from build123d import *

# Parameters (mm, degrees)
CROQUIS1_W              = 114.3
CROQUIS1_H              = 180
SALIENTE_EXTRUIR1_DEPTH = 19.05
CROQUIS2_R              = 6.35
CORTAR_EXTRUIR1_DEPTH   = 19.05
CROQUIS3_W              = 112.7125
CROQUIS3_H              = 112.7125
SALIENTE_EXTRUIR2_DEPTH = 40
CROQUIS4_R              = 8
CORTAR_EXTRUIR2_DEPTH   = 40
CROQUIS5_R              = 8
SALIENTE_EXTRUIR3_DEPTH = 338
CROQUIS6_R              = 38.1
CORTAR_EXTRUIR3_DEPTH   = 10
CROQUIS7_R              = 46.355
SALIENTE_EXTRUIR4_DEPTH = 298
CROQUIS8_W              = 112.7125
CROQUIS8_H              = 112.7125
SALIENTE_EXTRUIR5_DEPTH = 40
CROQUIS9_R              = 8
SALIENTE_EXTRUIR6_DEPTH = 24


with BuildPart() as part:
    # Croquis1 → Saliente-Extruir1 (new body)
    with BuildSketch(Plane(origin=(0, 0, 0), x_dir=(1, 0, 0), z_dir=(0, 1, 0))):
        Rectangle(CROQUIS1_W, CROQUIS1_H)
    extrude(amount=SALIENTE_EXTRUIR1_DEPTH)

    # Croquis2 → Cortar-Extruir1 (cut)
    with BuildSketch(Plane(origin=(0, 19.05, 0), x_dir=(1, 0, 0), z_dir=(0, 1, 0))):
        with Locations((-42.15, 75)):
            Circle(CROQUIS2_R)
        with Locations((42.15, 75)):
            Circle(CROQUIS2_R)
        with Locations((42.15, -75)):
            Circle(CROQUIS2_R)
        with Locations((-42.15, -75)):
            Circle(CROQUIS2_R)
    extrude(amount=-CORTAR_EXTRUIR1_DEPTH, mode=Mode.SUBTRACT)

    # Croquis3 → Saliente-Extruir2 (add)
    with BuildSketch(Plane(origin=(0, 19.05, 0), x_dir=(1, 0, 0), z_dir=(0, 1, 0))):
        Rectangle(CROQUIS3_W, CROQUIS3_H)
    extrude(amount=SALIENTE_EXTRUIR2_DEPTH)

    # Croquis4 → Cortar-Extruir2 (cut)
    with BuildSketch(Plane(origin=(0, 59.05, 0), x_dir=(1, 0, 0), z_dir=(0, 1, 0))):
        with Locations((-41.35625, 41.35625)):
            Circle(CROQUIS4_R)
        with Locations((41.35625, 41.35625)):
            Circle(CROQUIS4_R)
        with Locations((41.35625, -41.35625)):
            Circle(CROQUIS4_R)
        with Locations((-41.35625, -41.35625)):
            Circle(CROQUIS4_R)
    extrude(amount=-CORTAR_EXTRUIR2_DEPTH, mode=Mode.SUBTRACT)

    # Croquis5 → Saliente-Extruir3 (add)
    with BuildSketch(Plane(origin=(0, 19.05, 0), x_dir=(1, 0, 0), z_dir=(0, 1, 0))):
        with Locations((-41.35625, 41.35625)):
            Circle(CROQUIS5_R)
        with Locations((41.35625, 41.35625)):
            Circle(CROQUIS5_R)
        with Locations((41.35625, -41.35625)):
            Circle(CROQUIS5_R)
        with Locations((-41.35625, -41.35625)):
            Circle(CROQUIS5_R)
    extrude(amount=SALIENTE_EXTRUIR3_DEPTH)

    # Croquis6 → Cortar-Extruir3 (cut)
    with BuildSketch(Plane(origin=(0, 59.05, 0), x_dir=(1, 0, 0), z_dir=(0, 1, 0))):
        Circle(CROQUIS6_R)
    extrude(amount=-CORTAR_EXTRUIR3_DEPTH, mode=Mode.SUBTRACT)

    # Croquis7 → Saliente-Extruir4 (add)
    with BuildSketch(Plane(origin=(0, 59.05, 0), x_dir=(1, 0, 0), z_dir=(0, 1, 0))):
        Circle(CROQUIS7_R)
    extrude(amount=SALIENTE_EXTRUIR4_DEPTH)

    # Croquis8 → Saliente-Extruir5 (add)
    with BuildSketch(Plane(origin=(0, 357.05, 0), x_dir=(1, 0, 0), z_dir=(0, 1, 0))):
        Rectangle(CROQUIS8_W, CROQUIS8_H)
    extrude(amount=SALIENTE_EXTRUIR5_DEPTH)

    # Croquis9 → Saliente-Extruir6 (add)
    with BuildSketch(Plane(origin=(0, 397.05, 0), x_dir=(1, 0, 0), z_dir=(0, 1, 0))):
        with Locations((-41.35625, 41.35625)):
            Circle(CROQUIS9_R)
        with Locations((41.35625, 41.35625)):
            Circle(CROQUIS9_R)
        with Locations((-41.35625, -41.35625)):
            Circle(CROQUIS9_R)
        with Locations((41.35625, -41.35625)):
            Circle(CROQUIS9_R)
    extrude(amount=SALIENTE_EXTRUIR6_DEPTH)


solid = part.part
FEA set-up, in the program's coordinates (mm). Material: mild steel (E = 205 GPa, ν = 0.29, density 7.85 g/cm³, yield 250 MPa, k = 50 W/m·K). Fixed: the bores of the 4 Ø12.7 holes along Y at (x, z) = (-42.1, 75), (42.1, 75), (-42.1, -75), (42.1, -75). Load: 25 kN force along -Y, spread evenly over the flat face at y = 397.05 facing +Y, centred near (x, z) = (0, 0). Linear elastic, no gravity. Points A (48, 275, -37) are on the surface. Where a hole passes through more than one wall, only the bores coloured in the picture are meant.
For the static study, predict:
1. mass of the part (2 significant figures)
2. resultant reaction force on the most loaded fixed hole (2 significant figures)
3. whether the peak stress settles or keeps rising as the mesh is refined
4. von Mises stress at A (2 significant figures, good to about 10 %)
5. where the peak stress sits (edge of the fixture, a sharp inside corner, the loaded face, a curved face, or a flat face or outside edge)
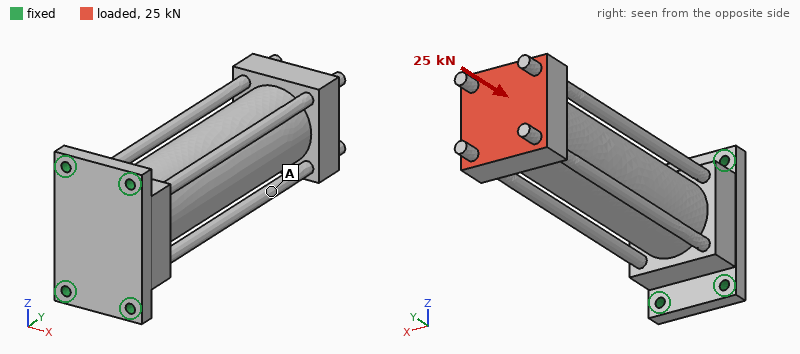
28 kg
6.9 kN
keeps rising
4.1 MPa
edge of the fixture
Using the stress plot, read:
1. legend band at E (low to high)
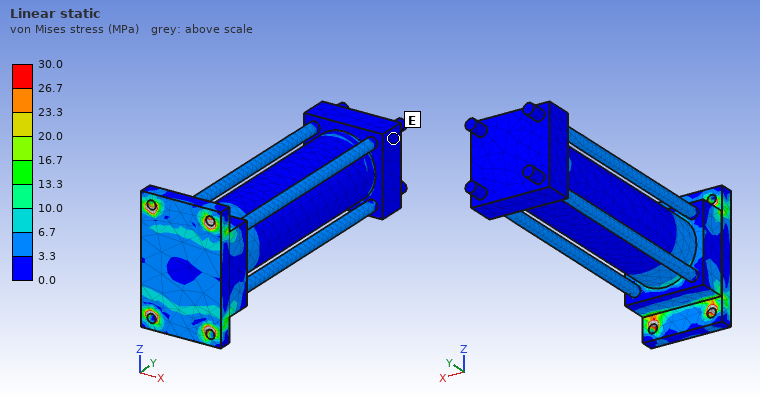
0.0 to 3.3 MPa
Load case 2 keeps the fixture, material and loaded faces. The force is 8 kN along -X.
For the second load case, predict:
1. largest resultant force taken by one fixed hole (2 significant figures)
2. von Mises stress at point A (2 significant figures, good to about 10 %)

19 kN
15 MPa
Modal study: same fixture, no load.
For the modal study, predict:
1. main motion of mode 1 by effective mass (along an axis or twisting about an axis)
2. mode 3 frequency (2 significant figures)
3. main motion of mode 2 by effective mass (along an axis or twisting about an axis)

along X
760 Hz
along Z
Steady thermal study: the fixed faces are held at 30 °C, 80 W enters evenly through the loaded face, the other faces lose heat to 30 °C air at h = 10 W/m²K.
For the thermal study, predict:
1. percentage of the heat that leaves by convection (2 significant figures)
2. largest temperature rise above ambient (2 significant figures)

64 %
50 K
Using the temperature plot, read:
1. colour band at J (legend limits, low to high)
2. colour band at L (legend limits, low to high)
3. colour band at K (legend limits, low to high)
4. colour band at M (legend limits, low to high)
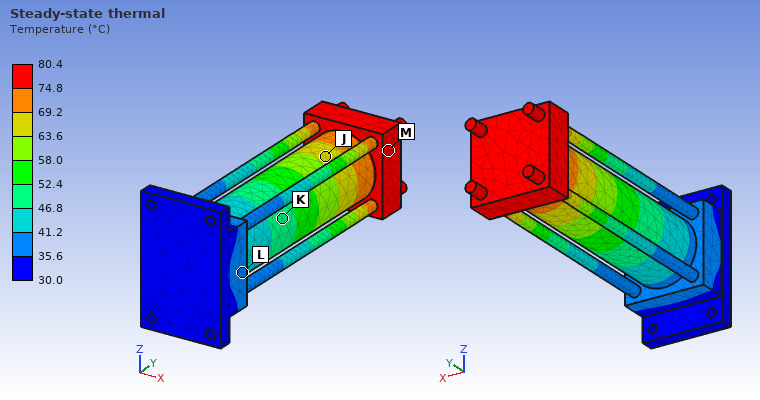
63.6 to 69.2 °C
35.6 to 41.2 °C
46.8 to 52.4 °C
74.8 to 80.4 °C
